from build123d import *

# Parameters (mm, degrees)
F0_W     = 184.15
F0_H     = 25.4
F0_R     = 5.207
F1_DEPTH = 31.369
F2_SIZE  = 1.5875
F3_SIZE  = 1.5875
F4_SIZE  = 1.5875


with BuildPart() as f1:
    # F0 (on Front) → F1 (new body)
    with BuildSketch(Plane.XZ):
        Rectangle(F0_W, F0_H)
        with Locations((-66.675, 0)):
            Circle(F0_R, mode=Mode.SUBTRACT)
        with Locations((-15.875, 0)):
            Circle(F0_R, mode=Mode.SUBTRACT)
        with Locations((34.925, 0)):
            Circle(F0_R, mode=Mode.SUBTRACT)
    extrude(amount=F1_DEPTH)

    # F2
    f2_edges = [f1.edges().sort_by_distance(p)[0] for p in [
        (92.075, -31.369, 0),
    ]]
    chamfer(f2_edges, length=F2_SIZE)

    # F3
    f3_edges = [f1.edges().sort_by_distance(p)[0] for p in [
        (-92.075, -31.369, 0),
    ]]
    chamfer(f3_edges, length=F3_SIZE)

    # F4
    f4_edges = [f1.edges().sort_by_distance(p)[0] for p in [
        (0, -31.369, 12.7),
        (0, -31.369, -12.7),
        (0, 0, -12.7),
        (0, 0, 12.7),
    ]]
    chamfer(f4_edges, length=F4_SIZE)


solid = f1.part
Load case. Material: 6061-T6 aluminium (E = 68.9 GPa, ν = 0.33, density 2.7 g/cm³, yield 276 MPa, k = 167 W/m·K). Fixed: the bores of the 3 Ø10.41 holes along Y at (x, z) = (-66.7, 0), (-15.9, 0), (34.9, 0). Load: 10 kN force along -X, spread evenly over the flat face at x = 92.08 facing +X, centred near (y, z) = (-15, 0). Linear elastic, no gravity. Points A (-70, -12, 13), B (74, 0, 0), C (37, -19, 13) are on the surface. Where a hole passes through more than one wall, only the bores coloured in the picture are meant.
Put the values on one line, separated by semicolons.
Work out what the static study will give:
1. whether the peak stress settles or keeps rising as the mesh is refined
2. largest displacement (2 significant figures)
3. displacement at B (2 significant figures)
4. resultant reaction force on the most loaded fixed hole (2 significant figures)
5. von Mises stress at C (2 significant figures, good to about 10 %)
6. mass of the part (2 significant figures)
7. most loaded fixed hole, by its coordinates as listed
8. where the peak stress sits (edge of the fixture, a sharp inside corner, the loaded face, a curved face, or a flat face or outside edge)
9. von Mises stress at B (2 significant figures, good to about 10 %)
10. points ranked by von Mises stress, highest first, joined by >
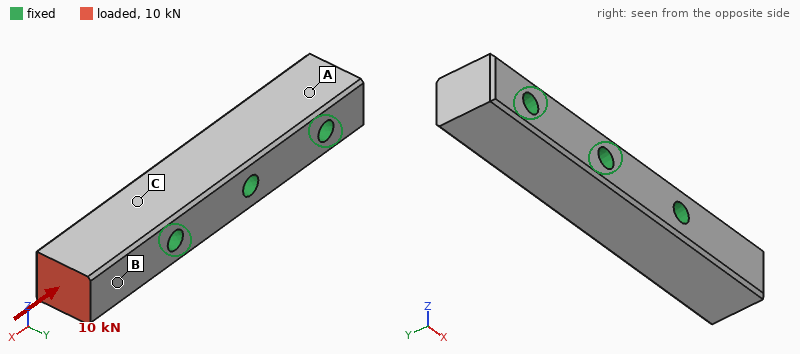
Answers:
keeps rising; 12 µm; 8.3 µm; 9.6 kN; 5.8 MPa; 370 g; (34.9, 0); edge of the fixture; 14 MPa; B > C > A
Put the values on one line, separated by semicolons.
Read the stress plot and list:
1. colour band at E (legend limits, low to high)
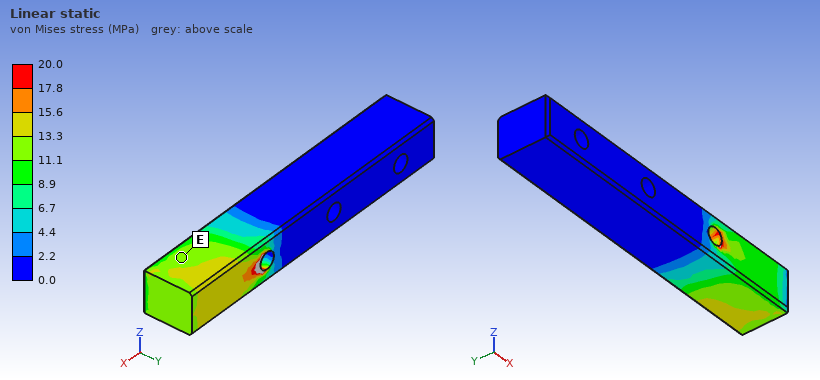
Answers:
11.1 to 13.3 MPa
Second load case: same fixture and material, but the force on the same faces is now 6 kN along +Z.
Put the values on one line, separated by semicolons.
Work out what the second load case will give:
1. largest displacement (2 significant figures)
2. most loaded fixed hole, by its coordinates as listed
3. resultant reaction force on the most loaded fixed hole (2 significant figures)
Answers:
0.18 mm; (34.9, 0); 8.1 kN
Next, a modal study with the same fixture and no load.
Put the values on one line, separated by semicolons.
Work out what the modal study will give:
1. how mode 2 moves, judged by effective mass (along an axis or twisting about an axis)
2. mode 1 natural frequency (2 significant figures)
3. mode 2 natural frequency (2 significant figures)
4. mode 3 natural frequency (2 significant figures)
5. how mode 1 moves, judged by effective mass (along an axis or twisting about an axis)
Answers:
along Y; 5100 Hz; 6900 Hz; 13 kHz; along Z
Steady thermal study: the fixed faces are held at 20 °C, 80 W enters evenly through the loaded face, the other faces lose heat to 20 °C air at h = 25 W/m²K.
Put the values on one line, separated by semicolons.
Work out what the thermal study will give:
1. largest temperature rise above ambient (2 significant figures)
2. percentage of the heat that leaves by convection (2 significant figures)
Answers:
33 K; 3.1 %
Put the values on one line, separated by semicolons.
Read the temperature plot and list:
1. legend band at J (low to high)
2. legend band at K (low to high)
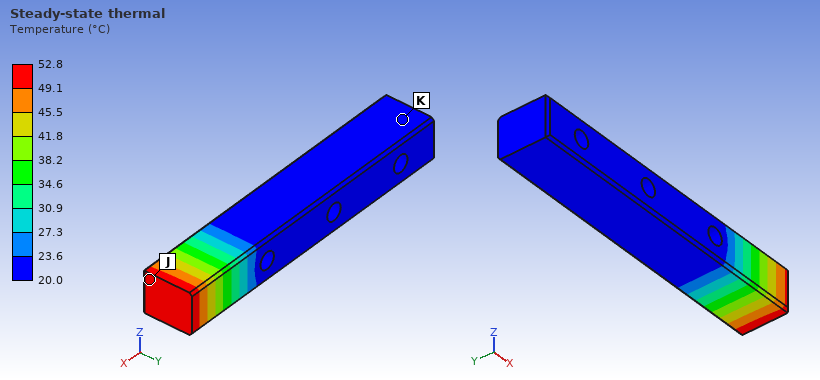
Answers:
49.1 to 52.8 °C; 20.0 to 23.6 °C
